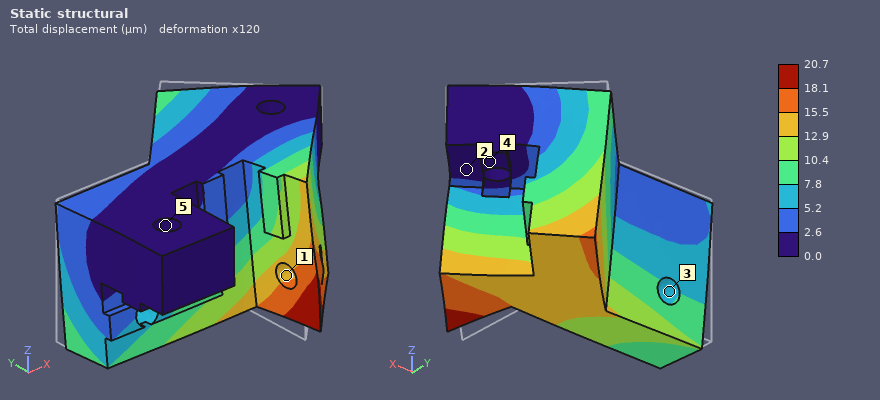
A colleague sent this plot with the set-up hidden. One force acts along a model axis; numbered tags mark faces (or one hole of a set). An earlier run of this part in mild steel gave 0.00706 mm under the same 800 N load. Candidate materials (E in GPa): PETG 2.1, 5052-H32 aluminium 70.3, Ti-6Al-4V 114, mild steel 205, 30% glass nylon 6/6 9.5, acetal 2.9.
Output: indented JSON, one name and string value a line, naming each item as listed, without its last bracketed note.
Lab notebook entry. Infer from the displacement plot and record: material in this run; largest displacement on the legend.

{
  "material in this run": "5052-H32 aluminium",
  "largest displacement on the legend": "20.7 µm"
}
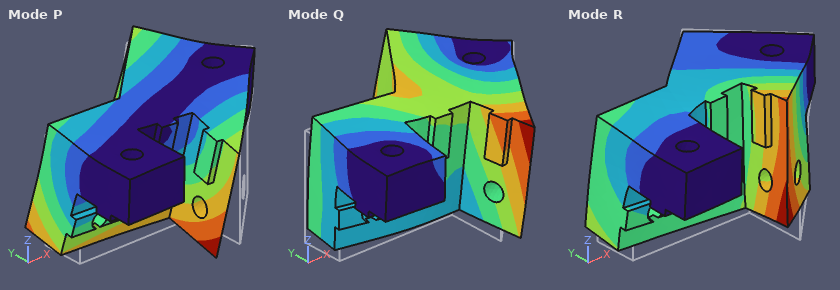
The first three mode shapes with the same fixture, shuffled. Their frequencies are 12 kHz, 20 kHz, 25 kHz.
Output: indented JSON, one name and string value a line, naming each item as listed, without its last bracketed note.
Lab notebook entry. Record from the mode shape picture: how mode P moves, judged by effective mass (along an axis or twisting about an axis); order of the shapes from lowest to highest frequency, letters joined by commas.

{
  "how mode P moves, judged by effective mass": "along Y",
  "order of the shapes from lowest to highest frequency, letters joined by commas": "P, R, Q"
}
